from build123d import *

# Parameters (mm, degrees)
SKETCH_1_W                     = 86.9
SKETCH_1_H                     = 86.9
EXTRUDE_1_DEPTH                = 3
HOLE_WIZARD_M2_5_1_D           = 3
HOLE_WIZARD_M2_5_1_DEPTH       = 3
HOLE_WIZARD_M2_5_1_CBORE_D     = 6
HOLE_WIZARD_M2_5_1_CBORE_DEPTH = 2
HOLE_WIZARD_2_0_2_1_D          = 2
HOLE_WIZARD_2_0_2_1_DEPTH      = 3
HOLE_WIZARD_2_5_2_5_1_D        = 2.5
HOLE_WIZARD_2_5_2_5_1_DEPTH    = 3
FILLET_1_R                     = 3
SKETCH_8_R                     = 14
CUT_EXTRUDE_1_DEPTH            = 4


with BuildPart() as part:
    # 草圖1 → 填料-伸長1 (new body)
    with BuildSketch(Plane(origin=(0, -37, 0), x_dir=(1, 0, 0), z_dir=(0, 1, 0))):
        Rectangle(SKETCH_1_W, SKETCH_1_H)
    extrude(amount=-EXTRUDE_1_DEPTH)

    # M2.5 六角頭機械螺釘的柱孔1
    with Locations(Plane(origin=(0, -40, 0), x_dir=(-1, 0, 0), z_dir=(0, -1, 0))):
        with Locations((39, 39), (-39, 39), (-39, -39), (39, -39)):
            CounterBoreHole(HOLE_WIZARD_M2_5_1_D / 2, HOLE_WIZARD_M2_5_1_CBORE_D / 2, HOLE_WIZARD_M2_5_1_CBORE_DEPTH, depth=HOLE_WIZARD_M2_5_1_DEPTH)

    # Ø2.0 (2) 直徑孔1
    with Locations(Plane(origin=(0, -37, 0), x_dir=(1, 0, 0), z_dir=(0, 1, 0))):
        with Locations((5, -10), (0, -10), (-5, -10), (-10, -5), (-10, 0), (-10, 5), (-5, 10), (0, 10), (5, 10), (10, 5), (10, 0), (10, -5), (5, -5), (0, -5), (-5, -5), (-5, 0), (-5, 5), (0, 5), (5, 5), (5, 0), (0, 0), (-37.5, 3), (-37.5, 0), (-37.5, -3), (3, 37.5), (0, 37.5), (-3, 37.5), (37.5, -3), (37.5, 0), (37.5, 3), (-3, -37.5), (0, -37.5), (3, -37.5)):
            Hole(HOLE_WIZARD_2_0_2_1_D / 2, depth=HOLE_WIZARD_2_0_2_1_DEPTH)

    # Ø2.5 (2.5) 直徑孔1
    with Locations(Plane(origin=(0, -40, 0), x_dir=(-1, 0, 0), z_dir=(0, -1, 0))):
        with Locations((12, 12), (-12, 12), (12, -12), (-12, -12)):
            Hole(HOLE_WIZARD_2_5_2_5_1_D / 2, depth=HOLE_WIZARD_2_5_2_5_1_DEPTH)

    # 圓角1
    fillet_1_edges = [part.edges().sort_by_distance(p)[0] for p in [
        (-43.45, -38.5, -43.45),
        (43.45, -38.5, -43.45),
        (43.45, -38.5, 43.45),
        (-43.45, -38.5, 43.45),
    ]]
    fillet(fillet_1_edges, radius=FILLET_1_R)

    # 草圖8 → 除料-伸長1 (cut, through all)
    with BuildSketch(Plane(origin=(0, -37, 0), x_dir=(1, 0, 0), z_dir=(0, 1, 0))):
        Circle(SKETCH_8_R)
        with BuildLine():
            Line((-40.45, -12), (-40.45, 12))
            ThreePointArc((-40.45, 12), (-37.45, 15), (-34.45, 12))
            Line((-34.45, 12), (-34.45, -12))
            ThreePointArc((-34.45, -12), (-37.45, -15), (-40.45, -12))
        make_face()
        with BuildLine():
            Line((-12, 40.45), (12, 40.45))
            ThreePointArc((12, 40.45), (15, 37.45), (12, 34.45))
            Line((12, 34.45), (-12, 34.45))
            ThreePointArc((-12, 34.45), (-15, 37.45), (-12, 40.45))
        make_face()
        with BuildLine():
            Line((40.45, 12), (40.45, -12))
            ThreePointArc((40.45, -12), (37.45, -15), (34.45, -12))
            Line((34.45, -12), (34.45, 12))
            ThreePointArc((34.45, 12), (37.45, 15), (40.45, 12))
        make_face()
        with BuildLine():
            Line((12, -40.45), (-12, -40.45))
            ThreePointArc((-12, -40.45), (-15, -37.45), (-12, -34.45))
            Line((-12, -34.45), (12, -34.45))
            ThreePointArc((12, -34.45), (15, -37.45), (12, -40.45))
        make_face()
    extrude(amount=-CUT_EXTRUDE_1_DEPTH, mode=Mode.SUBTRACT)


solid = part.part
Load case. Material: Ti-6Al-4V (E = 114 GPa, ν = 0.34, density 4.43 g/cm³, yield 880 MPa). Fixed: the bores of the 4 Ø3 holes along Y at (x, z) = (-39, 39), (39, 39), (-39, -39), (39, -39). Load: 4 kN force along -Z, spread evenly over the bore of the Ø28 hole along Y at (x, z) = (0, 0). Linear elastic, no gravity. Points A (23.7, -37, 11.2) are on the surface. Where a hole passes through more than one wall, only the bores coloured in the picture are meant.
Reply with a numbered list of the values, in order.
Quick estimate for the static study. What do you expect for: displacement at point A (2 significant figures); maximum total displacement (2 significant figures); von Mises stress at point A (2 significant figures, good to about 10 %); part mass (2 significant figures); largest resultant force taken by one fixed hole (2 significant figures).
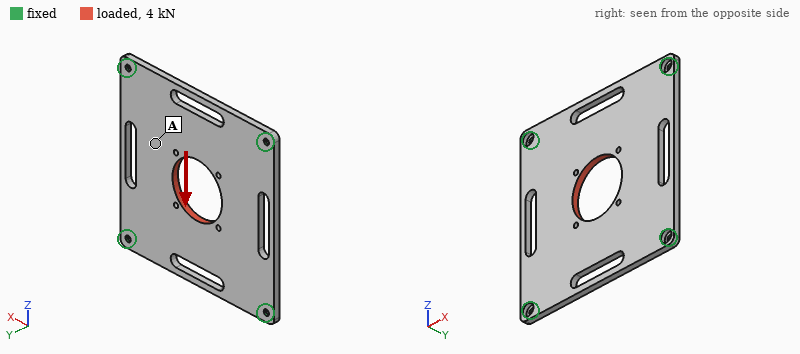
1. 14 µm
2. 23 µm
3. 18 MPa
4. 82 g
5. 1.1 kN
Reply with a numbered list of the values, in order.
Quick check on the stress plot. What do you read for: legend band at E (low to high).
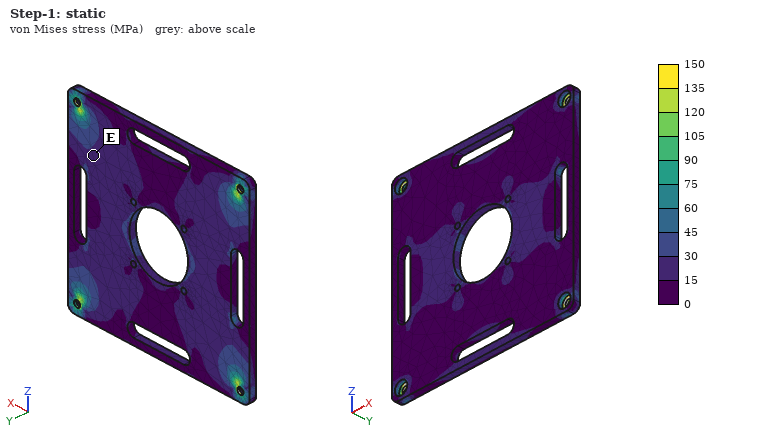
1. 15 to 30 MPa
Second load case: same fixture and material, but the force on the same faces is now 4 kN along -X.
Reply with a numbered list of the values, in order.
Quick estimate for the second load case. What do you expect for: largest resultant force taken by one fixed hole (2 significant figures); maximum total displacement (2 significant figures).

1. 1.1 kN
2. 23 µm
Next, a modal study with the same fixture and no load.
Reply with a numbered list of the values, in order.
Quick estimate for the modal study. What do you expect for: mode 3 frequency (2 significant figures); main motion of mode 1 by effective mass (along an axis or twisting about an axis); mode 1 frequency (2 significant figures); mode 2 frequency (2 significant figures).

1. 2300 Hz
2. along Y
3. 1300 Hz
4. 2300 Hz
